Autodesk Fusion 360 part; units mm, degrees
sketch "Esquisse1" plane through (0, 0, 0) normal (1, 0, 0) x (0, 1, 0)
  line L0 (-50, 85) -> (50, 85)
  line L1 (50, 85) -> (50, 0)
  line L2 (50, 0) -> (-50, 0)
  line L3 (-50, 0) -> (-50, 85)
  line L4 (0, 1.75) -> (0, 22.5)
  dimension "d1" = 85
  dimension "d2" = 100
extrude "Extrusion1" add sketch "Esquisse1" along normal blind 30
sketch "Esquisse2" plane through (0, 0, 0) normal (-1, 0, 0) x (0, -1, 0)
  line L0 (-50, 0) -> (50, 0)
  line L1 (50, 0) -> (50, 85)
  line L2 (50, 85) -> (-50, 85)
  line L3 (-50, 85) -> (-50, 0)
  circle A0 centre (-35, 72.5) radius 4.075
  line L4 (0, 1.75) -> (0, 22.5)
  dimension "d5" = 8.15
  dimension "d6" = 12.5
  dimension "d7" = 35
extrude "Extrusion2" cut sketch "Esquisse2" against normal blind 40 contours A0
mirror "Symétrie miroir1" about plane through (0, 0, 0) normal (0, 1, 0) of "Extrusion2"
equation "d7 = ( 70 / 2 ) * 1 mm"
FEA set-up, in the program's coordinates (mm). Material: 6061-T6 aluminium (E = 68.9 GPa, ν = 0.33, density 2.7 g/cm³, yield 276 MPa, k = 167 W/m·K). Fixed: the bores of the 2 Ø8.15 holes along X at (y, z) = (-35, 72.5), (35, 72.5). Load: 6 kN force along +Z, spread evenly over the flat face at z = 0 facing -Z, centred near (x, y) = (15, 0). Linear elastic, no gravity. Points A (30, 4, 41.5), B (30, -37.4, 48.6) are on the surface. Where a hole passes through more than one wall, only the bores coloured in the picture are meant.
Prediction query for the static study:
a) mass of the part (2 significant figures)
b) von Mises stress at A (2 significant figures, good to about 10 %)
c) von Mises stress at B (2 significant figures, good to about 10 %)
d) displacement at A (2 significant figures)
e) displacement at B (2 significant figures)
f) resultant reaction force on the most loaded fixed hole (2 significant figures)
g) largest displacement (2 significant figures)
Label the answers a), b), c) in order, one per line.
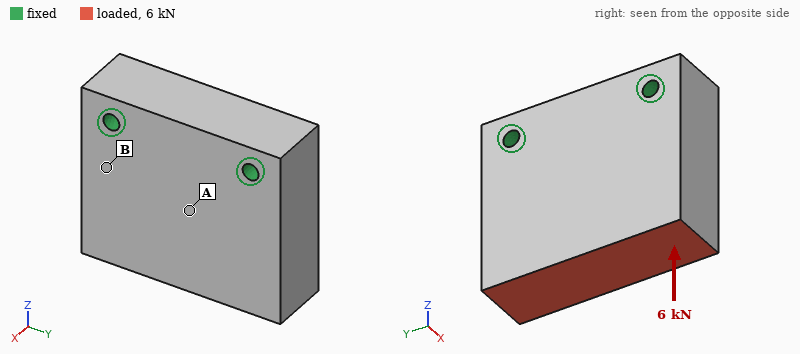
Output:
a) 680 g
b) 1.3 MPa
c) 2.7 MPa
d) 1.7 µm
e) 1.1 µm
f) 3.0 kN
g) 2.7 µm
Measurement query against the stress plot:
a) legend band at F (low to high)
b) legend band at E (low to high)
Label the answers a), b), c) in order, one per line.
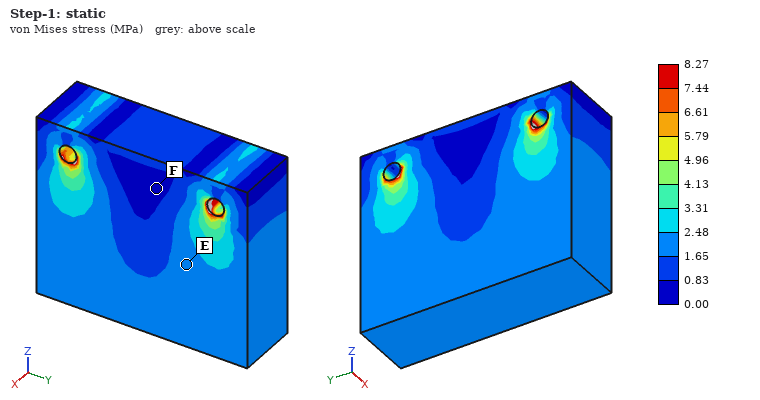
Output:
a) 0.00 to 0.83 MPa
b) 1.65 to 2.48 MPa
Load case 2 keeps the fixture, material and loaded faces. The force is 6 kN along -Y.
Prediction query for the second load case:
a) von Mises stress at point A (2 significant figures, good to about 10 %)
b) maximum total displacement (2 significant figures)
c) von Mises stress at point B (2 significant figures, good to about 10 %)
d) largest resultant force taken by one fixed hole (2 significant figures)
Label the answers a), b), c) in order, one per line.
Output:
a) 5.5 MPa
b) 15 µm
c) 5.0 MPa
d) 6.6 kN
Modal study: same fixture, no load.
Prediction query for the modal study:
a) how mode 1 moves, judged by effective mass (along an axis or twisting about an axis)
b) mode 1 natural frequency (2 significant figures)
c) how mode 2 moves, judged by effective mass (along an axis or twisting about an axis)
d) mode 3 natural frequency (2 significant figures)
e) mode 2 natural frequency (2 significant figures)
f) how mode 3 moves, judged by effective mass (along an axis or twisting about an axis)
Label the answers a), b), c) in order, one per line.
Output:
a) along X
b) 3400 Hz
c) twisting about Z
d) 7500 Hz
e) 6700 Hz
f) along Y
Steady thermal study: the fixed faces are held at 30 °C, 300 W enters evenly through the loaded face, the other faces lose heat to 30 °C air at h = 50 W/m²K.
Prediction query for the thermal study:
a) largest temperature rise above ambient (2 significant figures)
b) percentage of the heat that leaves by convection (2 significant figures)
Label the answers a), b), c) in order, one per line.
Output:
a) 46 K
b) 8.1 %
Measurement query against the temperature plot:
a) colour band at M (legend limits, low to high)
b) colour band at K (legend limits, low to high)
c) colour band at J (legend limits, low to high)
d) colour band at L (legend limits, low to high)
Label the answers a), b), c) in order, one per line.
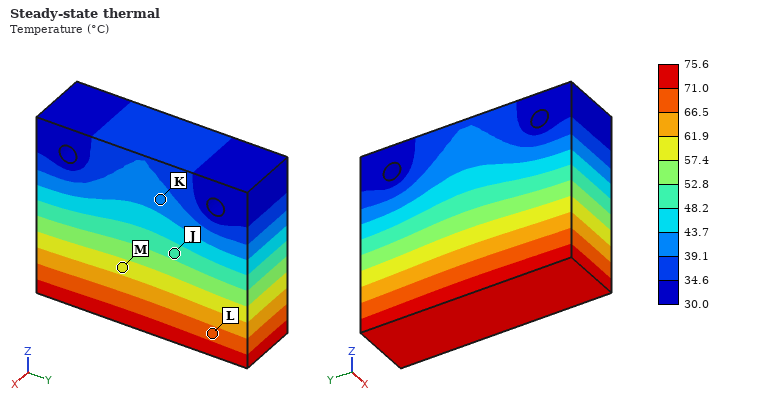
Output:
a) 57.4 to 61.9 °C
b) 39.1 to 43.7 °C
c) 48.2 to 52.8 °C
d) 66.5 to 71.0 °C
